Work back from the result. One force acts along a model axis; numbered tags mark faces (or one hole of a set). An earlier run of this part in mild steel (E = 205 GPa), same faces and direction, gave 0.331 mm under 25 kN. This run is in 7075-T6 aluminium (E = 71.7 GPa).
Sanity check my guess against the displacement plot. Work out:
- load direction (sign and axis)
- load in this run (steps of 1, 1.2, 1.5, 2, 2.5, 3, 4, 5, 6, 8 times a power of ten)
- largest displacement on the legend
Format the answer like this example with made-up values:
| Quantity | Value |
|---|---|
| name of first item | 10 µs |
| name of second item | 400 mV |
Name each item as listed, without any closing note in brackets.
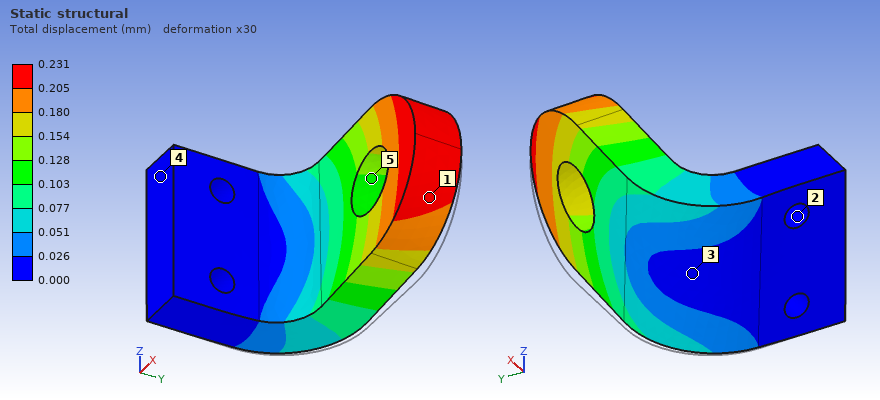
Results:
| Quantity | Value |
|---|---|
| load direction | +Z |
| load in this run | 6 kN |
| largest displacement on the legend | 0.231 mm |
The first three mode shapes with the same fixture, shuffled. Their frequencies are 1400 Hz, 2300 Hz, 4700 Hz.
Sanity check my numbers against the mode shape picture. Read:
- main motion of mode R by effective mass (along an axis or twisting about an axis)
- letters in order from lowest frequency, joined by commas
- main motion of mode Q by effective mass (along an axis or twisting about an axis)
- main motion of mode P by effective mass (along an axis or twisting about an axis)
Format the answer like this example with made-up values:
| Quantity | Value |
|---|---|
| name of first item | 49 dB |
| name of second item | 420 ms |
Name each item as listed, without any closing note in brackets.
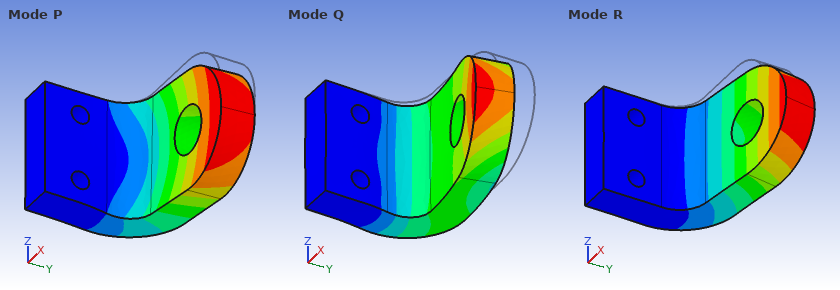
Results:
| Quantity | Value |
|---|---|
| main motion of mode R by effective mass | along Y |
| letters in order from lowest frequency, joined by commas | R, P, Q |
| main motion of mode Q by effective mass | along X |
| main motion of mode P by effective mass | along Z |
